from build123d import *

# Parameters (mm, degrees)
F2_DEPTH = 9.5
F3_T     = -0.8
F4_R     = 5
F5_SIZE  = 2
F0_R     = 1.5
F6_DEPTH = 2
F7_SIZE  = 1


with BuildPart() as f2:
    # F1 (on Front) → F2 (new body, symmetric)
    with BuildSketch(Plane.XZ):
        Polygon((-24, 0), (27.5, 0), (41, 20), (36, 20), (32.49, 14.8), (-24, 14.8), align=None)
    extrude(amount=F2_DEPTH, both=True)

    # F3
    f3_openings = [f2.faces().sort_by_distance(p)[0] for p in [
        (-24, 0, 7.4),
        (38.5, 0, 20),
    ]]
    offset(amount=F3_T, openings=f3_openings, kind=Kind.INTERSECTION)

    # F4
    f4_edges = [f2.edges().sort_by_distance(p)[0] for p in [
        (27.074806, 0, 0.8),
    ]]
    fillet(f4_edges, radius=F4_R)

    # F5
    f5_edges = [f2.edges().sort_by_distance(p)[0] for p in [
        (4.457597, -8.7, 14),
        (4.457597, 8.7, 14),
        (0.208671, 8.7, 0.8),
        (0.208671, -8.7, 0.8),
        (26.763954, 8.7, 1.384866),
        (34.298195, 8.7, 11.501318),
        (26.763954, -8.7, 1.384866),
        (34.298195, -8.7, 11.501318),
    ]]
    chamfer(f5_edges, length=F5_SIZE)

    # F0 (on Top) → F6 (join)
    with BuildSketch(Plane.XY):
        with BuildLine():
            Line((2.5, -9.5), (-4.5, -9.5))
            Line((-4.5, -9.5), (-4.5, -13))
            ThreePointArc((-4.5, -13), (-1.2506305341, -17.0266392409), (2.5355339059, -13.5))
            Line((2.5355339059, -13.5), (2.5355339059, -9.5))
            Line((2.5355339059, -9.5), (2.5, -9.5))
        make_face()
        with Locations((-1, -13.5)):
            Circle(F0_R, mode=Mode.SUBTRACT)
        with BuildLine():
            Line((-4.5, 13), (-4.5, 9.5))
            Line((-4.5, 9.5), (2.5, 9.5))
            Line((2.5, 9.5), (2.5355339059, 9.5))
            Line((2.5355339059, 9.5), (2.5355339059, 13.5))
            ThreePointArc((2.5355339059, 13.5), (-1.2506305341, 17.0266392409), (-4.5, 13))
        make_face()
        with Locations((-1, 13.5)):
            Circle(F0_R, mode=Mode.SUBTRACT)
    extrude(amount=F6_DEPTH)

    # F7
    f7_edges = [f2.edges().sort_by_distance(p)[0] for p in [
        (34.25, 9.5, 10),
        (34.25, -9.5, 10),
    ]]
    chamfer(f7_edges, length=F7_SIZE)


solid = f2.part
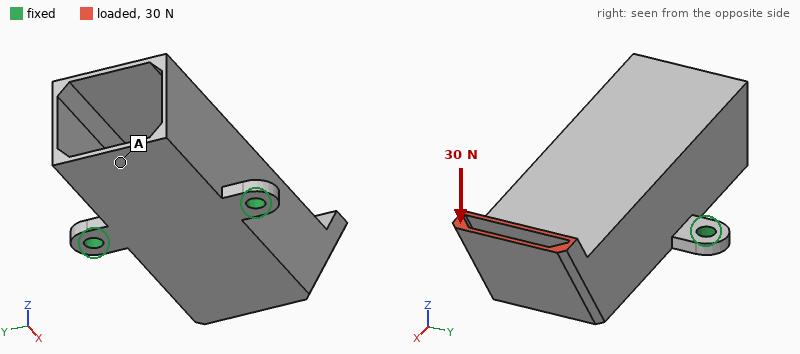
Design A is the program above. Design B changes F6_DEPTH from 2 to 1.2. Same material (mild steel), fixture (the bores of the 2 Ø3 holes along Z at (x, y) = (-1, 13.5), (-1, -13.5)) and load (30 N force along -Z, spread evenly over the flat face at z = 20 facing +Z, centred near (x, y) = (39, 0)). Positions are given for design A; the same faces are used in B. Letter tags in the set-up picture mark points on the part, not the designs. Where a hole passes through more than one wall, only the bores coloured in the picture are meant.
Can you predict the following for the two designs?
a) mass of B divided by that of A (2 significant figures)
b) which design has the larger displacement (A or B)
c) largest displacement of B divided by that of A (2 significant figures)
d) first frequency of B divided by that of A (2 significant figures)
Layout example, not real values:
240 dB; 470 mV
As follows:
0.98; B; 2.8; 0.59
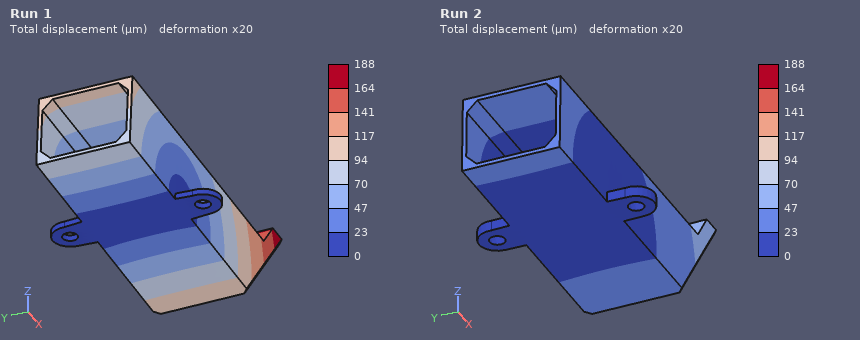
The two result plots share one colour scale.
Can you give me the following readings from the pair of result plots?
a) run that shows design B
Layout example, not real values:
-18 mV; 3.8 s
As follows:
Run 1
